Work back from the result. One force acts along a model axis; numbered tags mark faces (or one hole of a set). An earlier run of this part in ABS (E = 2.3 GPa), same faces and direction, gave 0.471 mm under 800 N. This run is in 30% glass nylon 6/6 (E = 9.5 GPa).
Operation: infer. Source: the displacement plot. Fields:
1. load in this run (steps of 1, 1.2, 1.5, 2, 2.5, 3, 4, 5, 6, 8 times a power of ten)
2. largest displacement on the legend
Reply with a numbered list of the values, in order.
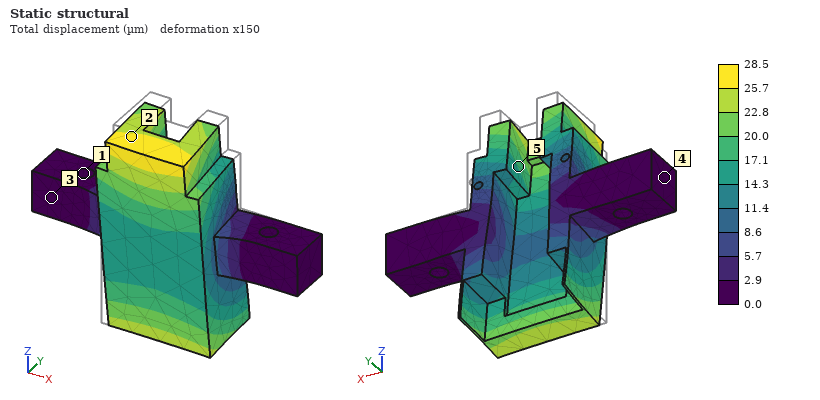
1. 200 N
2. 28.5 µm
